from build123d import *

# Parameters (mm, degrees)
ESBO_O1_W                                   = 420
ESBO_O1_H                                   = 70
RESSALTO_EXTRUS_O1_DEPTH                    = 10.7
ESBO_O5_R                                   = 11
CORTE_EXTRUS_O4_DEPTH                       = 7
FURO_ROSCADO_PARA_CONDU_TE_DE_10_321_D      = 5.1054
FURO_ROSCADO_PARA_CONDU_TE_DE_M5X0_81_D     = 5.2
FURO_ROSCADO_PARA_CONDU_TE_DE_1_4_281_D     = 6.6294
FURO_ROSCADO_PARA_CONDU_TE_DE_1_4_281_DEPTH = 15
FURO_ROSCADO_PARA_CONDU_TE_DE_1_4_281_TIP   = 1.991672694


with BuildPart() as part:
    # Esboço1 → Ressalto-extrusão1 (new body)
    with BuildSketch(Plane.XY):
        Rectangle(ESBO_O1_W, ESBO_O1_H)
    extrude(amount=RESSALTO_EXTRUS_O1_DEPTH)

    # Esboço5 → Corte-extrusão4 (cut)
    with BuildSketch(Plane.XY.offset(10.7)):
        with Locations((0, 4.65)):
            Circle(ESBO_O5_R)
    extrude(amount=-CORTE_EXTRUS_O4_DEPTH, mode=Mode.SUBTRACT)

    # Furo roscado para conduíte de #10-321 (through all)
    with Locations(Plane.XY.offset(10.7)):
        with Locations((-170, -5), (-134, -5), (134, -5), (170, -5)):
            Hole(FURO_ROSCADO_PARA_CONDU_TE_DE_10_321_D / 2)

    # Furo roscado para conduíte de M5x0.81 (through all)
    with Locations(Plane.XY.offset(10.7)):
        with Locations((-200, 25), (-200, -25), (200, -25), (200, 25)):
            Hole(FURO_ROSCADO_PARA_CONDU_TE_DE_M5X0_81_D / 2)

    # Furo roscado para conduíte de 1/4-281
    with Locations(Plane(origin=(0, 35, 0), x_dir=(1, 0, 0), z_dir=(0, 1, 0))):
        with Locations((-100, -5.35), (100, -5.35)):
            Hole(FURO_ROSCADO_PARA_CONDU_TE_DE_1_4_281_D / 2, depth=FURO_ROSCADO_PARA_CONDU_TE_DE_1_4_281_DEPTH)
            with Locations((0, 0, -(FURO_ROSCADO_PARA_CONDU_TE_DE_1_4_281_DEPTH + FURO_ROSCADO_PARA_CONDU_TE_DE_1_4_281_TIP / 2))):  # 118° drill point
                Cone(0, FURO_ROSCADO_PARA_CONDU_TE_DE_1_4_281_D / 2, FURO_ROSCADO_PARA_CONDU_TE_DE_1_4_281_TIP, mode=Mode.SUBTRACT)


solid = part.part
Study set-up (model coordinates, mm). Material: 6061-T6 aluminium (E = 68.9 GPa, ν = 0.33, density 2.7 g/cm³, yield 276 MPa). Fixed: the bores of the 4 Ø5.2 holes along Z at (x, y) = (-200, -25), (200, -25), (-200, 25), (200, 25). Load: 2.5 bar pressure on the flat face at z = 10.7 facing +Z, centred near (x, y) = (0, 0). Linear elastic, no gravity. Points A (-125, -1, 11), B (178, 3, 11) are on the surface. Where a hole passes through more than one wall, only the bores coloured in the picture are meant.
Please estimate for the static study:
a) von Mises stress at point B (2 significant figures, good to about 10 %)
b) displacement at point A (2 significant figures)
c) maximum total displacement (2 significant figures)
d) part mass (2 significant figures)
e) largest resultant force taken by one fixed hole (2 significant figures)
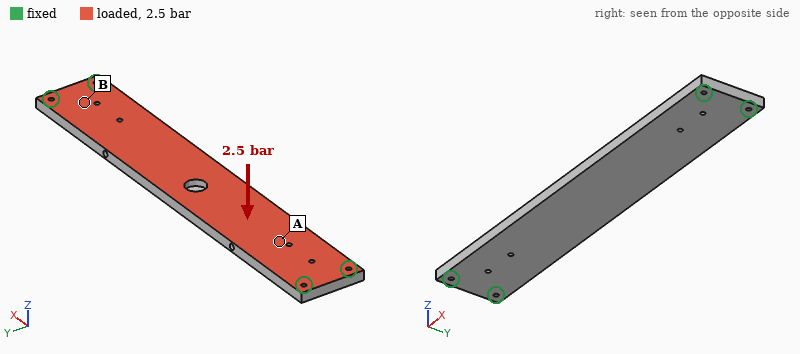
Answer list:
100 MPa
1.0 mm
2.6 mm
830 g
1.8 kN
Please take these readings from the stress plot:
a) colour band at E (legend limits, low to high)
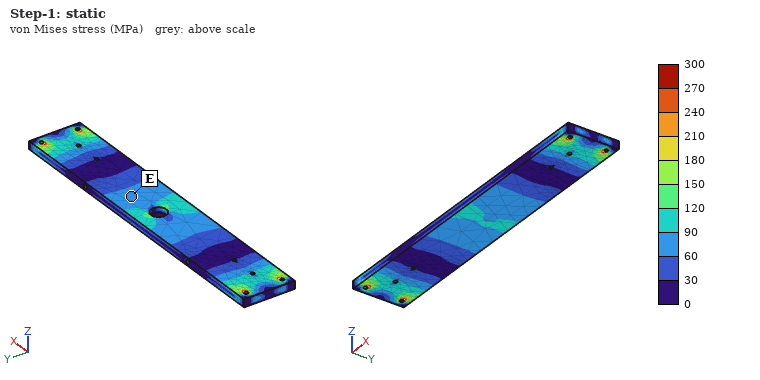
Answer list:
60 to 90 MPa
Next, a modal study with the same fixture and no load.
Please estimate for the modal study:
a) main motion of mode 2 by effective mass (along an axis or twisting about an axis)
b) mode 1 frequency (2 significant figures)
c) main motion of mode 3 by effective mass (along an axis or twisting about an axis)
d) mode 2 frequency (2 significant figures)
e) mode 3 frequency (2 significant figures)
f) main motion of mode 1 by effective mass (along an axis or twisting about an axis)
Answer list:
twisting about Y
330 Hz
twisting about X
920 Hz
1200 Hz
along Z
